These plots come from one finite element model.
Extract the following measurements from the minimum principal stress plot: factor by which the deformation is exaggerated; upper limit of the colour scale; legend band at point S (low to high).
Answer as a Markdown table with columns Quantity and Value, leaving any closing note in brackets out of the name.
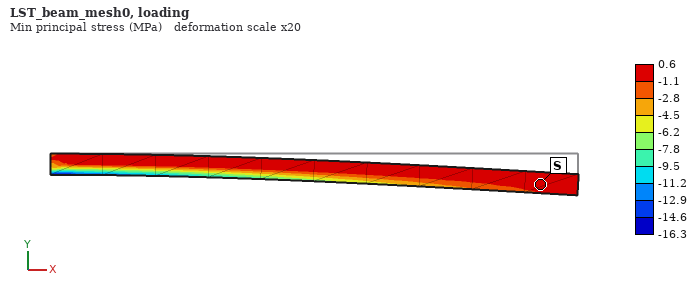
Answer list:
| Quantity | Value |
|---|---|
| factor by which the deformation is exaggerated | 20 |
| upper limit of the colour scale | 0.6 MPa |
| legend band at point S | -1.1 to 0.6 MPa |
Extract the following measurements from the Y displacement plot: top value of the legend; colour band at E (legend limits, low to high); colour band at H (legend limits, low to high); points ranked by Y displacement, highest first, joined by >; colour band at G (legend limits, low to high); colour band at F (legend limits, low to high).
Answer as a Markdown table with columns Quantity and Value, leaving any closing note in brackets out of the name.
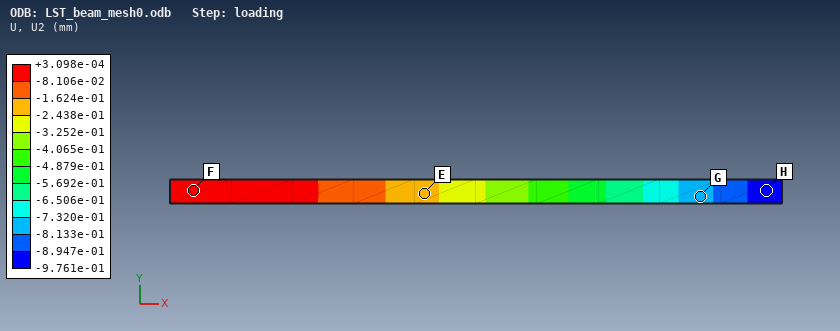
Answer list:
| Quantity | Value |
|---|---|
| top value of the legend | +3.098e-04 mm |
| colour band at E | -2.438e-01 to -1.624e-01 mm |
| colour band at H | -9.761e-01 to -8.947e-01 mm |
| points ranked by Y displacement, highest first, joined by > | F > E > G > H |
| colour band at G | -8.133e-01 to -7.320e-01 mm |
| colour band at F | -8.106e-02 to +3.098e-04 mm |
